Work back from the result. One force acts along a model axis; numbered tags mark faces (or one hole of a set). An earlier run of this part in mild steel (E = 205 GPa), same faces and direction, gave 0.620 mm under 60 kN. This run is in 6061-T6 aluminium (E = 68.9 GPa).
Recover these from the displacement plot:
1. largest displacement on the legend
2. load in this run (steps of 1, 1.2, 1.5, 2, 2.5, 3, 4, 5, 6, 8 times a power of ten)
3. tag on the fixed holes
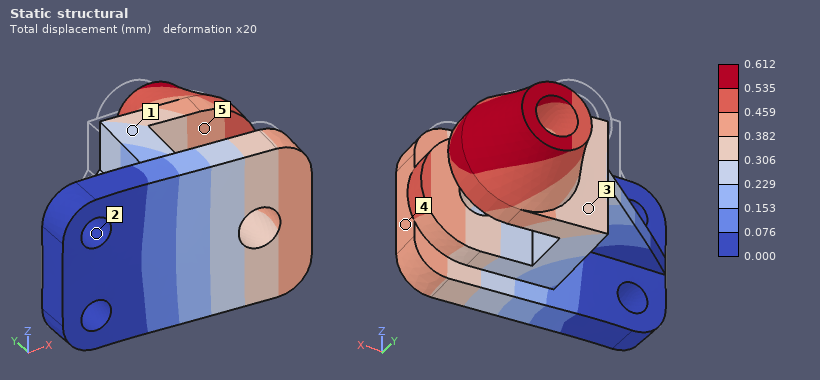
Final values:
0.612 mm
20 kN
2
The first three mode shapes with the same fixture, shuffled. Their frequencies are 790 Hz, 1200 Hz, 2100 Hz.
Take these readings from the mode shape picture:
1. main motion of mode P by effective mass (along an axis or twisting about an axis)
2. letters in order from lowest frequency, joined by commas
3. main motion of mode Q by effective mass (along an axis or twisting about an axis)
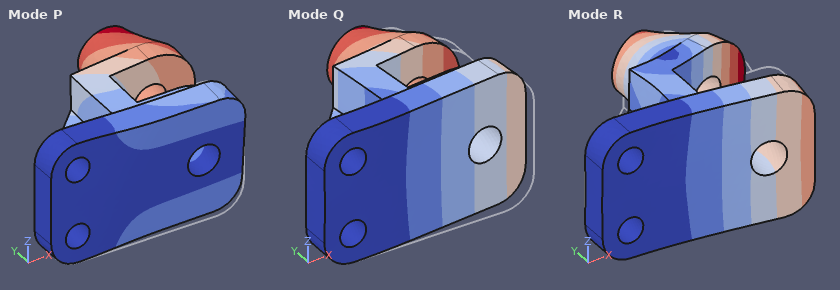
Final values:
along Z
Q, P, R
along Y
